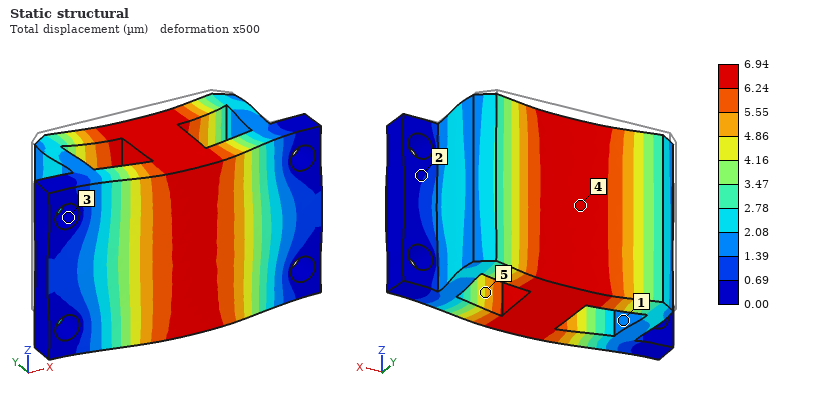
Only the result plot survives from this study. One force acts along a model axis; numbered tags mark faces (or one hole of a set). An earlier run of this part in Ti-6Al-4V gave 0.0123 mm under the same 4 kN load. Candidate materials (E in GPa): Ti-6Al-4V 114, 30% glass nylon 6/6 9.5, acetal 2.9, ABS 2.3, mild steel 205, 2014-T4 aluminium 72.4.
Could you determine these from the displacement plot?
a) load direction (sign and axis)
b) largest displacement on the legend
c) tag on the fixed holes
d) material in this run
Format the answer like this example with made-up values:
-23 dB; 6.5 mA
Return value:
-Y; 6.94 µm; 3; mild steel
